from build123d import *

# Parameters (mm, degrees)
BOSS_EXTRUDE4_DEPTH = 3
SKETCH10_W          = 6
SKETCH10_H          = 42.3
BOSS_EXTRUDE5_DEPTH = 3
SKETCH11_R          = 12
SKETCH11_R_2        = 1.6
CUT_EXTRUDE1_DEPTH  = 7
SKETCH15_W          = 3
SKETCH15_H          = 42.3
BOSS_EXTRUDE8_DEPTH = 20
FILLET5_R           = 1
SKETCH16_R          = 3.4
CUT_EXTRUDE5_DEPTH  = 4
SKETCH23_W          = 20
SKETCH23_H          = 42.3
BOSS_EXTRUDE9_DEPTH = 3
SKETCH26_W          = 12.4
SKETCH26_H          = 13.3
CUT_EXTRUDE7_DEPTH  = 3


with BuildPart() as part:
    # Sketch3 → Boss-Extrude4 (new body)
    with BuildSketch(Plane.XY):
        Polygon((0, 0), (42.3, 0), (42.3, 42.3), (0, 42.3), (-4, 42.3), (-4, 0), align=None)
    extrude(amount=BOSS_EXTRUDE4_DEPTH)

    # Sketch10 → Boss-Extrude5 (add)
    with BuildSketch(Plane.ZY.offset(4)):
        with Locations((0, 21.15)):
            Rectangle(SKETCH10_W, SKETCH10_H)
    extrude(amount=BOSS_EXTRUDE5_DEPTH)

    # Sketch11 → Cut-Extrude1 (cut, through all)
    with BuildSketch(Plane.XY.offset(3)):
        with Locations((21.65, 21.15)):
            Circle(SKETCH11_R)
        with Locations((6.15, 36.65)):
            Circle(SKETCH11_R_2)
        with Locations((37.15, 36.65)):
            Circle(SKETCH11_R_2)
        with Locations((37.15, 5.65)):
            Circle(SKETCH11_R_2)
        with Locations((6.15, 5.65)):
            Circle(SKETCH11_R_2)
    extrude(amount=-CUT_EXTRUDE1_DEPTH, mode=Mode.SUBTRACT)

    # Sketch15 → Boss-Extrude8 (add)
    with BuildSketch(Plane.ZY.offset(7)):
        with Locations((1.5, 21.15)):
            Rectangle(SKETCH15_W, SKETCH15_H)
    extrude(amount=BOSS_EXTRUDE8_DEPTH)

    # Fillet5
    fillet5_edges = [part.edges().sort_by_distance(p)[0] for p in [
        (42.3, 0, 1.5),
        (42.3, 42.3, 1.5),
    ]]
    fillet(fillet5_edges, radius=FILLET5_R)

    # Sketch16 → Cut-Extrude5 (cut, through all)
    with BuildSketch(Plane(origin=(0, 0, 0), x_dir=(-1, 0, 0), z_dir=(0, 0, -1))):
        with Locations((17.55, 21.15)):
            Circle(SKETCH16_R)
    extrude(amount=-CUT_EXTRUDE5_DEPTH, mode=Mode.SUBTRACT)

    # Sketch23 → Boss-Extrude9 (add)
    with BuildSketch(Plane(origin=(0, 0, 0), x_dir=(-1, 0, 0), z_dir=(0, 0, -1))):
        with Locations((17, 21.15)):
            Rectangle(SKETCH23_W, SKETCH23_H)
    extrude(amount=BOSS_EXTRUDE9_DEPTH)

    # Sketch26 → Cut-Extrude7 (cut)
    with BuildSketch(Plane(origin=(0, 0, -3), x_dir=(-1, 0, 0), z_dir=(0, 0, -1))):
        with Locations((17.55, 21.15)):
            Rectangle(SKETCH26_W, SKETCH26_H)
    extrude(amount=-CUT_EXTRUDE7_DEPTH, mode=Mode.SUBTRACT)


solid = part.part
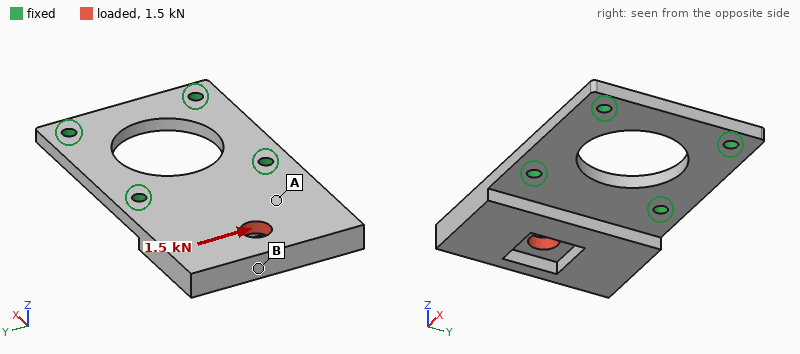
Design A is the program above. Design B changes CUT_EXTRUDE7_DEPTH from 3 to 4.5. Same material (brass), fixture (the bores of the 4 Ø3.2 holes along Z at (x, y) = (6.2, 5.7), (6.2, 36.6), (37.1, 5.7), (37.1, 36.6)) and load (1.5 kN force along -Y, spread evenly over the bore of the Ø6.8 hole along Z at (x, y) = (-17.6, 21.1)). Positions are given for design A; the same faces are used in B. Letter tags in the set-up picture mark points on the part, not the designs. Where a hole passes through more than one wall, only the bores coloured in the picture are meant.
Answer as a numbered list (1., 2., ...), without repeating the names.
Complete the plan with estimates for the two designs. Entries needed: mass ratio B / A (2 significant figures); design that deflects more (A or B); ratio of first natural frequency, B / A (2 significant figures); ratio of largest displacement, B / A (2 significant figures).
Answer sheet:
1. 0.98
2. B
3. 1.0
4. 1.3
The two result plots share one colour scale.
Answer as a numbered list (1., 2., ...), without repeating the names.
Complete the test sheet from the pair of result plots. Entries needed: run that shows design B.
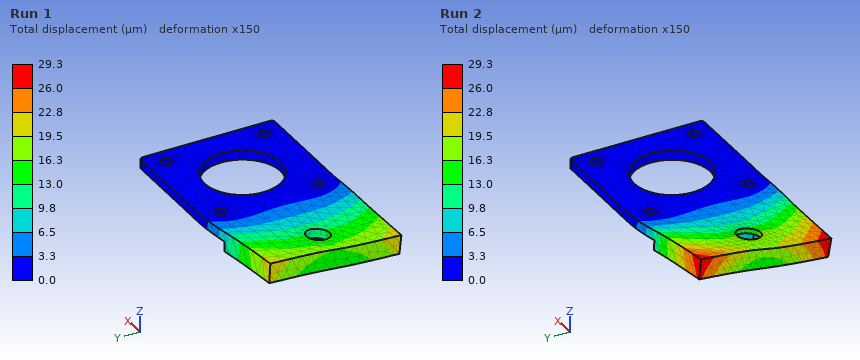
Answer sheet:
1. Run 2
